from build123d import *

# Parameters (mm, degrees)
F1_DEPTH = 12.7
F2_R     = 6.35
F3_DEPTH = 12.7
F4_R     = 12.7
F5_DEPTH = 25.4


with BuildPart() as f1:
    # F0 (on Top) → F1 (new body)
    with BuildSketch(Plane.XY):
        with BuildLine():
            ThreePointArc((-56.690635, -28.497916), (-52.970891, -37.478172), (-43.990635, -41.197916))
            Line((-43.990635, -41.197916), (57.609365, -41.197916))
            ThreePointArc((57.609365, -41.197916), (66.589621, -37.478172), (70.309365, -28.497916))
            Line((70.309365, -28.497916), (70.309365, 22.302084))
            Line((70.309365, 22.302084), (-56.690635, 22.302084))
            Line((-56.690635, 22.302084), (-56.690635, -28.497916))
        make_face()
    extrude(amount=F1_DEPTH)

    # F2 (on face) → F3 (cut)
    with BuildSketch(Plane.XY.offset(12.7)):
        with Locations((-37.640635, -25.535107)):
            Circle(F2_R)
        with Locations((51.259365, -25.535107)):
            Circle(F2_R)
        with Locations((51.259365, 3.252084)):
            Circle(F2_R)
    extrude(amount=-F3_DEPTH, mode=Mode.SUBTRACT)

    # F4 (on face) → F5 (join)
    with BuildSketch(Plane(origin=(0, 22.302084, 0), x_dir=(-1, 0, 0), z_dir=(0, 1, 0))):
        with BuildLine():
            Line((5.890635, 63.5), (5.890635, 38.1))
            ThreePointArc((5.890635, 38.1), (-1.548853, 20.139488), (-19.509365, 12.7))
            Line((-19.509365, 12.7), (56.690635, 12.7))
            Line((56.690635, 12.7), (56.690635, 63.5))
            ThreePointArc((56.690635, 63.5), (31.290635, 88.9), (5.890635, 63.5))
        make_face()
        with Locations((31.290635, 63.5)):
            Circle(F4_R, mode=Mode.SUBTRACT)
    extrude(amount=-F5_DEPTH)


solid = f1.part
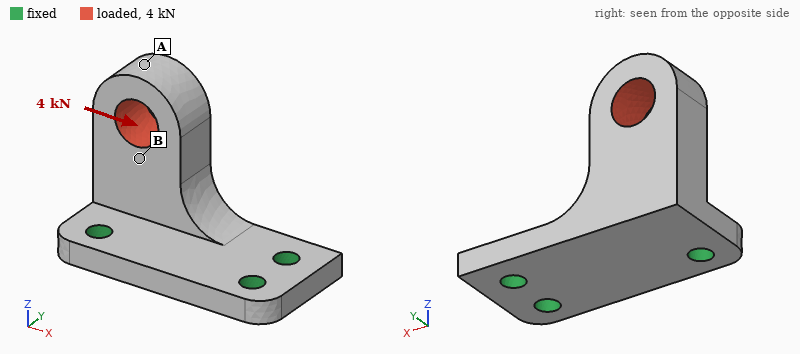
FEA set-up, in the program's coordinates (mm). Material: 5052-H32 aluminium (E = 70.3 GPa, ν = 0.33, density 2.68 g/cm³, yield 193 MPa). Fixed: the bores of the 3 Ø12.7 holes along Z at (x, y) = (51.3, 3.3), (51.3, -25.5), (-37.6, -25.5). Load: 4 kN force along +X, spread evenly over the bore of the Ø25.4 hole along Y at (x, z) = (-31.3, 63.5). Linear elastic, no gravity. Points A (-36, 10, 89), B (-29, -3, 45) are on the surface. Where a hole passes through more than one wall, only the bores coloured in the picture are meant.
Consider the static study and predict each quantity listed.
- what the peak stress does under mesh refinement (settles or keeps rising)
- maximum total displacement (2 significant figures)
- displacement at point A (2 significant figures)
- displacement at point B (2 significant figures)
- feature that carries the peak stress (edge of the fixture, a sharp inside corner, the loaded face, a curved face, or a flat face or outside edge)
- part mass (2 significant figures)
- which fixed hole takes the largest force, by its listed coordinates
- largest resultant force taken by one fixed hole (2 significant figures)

keeps rising
0.16 mm
0.16 mm
0.071 mm
edge of the fixture
480 g
(-37.6, -25.5)
3.0 kN
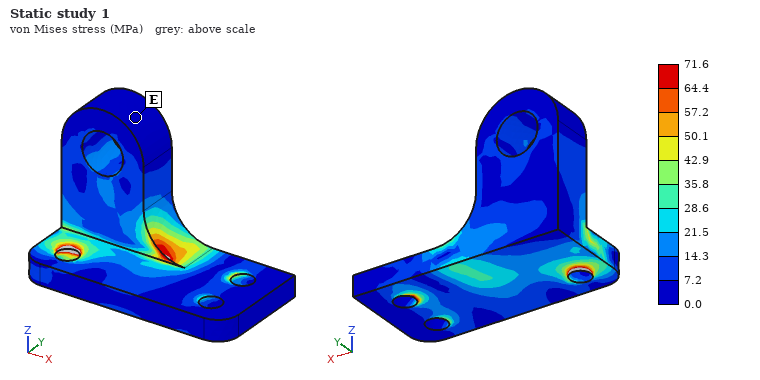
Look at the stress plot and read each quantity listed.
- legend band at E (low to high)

0.0 to 7.2 MPa
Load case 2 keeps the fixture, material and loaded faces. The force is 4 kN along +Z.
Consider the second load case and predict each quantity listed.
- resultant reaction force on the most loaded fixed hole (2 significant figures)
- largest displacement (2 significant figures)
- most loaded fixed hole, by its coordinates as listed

3.4 kN
0.17 mm
(-37.6, -25.5)
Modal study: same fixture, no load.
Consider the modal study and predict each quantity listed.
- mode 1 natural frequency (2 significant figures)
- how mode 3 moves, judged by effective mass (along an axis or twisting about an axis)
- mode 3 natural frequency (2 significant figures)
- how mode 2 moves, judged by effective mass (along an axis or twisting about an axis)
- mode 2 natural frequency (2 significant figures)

1300 Hz
along Z
4700 Hz
along X
2800 Hz
